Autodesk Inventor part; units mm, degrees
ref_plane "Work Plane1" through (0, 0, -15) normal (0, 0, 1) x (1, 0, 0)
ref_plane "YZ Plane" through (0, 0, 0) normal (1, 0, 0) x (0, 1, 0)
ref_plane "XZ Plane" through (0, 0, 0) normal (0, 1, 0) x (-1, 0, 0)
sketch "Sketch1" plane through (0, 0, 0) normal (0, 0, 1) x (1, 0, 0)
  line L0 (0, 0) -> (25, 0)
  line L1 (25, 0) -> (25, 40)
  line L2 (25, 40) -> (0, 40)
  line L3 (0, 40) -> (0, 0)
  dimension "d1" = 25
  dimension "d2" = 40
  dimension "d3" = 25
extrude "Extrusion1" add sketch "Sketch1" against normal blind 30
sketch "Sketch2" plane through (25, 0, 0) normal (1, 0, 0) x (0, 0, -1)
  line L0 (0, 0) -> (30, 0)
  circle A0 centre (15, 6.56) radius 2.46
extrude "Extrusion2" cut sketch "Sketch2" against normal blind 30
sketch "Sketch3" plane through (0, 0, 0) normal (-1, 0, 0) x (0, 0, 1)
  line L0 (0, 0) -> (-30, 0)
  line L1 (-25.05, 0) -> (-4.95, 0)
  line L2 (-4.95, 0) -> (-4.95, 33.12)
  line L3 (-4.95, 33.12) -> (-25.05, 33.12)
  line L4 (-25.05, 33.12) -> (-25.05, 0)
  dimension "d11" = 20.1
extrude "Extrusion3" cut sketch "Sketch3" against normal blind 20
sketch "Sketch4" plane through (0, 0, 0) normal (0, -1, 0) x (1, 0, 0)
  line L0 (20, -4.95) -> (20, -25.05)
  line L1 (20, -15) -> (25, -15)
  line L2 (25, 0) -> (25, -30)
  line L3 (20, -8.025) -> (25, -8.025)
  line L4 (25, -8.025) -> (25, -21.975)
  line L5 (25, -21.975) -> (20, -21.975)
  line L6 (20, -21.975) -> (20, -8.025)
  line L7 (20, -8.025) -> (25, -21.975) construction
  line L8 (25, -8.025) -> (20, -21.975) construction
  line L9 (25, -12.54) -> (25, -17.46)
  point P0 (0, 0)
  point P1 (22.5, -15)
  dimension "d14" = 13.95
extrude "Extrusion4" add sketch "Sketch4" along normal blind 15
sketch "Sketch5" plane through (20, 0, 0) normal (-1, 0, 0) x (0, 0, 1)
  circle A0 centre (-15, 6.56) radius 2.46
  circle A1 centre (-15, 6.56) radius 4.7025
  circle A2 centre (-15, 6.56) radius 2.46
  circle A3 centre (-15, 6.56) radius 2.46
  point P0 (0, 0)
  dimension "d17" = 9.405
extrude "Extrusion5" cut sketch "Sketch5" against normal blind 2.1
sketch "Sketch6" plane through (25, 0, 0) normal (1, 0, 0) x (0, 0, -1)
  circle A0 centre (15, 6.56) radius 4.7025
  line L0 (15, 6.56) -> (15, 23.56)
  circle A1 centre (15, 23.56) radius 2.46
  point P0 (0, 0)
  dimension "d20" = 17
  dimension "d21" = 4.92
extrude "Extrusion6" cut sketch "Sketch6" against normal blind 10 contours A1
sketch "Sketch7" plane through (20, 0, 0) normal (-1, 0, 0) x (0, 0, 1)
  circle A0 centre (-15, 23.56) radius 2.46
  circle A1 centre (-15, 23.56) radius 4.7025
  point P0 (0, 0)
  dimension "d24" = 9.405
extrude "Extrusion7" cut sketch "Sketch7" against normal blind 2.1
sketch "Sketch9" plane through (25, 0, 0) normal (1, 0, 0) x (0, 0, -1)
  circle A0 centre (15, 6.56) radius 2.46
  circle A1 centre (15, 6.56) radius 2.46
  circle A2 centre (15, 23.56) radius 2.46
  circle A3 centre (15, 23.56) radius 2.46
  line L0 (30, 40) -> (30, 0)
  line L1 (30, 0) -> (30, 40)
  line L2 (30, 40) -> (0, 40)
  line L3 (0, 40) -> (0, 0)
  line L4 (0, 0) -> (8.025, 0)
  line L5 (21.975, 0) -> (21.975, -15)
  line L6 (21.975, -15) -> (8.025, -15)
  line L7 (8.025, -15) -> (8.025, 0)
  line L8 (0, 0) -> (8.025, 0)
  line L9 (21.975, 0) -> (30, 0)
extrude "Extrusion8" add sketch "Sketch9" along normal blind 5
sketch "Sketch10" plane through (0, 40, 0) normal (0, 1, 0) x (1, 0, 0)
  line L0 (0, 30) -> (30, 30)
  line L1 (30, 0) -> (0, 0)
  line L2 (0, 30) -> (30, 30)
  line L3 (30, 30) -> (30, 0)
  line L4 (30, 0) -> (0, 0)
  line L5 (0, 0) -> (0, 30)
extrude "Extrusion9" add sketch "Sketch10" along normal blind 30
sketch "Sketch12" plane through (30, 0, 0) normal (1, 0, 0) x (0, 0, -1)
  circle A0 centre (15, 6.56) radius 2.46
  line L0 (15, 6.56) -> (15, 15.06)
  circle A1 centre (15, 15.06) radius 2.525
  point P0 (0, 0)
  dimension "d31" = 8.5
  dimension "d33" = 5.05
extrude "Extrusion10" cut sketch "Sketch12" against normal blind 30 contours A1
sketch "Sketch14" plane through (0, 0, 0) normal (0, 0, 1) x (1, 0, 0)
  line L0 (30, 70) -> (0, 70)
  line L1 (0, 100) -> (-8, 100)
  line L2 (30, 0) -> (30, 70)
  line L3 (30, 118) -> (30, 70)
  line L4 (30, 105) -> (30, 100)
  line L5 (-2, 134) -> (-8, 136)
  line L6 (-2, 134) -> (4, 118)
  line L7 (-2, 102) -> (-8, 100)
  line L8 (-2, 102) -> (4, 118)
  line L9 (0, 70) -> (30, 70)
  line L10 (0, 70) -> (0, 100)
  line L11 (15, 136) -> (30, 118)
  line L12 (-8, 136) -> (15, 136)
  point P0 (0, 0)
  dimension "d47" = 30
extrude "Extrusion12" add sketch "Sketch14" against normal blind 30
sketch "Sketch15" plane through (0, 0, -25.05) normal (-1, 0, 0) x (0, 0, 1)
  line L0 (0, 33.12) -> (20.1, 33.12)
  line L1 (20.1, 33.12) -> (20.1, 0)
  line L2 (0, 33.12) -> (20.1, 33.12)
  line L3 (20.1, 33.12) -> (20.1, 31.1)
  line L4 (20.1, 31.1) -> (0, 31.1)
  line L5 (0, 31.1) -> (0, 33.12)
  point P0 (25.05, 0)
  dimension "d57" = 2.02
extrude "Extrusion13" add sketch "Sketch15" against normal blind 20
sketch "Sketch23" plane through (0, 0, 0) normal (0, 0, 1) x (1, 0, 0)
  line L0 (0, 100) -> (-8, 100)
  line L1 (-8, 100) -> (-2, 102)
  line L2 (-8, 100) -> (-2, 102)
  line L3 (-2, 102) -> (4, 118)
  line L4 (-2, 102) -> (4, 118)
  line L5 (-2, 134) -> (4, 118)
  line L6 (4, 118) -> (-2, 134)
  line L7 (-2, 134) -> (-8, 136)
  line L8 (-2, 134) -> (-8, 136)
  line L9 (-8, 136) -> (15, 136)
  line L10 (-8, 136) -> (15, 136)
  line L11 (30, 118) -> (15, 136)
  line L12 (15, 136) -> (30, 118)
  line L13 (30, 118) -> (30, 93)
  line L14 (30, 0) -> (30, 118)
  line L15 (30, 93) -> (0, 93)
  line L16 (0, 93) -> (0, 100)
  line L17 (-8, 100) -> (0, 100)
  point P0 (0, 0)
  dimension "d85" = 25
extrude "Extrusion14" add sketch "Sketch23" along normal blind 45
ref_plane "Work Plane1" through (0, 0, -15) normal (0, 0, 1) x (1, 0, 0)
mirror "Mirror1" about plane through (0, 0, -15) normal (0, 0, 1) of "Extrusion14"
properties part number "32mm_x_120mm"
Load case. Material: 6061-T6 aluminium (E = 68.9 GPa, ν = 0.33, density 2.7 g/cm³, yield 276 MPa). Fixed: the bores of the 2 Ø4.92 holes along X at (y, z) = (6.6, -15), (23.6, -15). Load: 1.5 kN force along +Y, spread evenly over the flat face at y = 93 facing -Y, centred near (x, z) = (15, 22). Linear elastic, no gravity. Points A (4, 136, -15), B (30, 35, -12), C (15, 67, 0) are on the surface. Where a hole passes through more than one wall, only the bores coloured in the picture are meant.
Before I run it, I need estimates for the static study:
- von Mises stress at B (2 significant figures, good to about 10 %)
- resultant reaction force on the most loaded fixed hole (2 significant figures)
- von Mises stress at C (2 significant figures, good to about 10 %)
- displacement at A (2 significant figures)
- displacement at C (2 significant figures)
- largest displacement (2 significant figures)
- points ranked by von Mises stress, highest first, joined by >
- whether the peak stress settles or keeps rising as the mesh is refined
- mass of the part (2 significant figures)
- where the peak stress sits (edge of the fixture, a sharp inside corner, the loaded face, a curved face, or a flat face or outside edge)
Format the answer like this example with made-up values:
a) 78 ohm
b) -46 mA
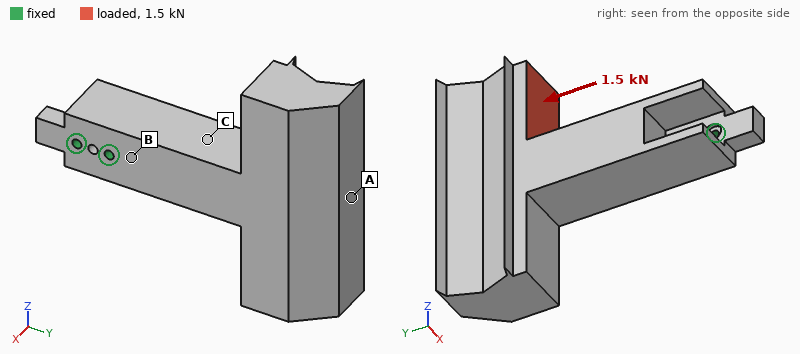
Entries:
a) 8.1 MPa
b) 2.7 kN
c) 14 MPa
d) 0.16 mm
e) 0.053 mm
f) 0.21 mm
g) C > B > A
h) keeps rising
i) 570 g
j) edge of the fixture
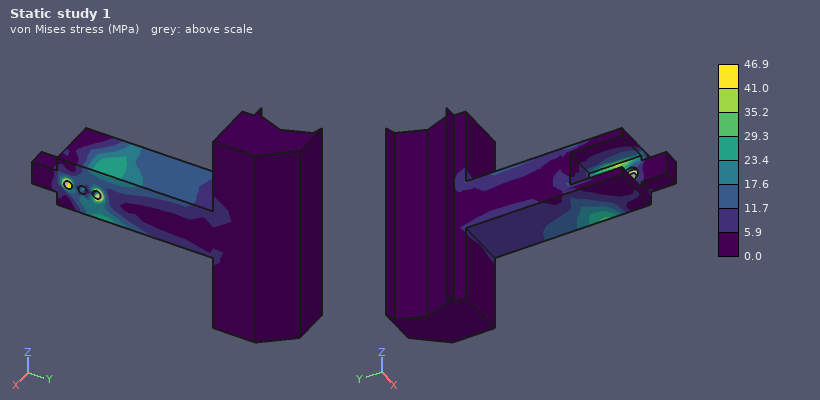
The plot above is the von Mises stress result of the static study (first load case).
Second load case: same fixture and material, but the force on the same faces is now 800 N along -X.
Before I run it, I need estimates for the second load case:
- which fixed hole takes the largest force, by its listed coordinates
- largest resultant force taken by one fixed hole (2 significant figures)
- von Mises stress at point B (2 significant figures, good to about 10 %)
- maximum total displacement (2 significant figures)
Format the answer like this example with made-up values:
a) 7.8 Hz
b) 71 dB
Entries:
a) (23.6, -15)
b) 3.0 kN
c) 19 MPa
d) 0.30 mm
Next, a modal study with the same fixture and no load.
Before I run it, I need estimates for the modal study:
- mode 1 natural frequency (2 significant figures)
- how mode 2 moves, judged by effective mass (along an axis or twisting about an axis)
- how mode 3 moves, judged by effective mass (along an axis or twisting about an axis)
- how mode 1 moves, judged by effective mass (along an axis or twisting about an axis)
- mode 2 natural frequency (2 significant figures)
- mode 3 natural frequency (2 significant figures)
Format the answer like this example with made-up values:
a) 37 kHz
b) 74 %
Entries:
a) 520 Hz
b) along Z
c) twisting about Y
d) along X
e) 570 Hz
f) 850 Hz
